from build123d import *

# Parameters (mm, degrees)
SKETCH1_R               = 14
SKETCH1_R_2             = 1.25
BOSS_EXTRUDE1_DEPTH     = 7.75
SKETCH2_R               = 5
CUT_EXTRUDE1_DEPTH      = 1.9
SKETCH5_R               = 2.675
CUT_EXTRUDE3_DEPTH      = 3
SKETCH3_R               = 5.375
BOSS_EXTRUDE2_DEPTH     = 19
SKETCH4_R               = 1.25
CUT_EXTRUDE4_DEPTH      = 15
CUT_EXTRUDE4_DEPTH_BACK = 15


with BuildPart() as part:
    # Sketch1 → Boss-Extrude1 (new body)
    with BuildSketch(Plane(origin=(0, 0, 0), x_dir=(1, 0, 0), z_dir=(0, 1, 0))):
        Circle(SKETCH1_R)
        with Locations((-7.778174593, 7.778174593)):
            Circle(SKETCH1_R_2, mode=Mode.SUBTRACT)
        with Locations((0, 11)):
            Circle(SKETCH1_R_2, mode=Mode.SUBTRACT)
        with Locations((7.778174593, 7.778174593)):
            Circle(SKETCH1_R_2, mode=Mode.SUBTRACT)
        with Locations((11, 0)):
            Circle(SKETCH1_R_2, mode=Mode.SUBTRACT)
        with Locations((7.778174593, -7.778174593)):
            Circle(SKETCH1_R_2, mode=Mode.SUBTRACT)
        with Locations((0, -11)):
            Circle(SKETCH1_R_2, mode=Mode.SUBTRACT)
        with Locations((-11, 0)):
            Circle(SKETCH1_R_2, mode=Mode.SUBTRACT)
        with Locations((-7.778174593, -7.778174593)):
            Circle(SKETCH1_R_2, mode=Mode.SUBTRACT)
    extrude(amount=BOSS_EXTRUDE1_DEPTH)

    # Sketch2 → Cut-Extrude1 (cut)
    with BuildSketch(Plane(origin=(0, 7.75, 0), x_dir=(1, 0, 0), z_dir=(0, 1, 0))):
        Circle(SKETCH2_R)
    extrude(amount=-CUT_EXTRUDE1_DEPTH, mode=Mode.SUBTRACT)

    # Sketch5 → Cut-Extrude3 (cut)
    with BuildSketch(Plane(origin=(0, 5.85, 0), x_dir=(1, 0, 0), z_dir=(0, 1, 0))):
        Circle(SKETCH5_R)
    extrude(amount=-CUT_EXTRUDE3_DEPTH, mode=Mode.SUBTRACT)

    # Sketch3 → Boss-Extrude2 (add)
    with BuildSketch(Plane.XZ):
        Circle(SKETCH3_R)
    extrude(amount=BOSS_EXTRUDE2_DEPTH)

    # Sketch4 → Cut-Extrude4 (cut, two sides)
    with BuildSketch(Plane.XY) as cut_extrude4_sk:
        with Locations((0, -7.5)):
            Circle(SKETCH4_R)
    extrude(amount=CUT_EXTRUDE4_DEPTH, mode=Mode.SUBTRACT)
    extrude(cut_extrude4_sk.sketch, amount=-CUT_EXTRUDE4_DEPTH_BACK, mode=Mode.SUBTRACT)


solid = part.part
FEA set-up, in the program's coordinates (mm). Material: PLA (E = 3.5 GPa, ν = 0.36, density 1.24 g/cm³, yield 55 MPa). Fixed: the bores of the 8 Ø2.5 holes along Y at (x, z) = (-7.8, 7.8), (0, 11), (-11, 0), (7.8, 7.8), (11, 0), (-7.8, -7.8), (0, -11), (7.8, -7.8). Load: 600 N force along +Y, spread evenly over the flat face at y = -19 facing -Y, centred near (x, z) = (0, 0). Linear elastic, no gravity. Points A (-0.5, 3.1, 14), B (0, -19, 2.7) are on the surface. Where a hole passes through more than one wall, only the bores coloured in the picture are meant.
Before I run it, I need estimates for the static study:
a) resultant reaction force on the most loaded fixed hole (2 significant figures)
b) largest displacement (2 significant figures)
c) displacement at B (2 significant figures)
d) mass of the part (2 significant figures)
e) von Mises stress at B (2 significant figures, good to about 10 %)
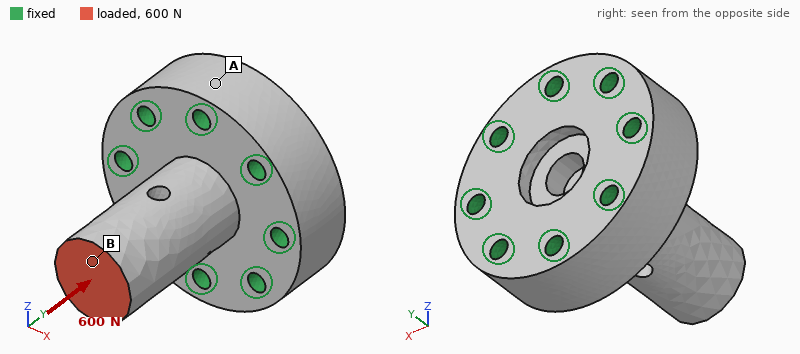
91 N
54 µm
54 µm
7.3 g
6.5 MPa
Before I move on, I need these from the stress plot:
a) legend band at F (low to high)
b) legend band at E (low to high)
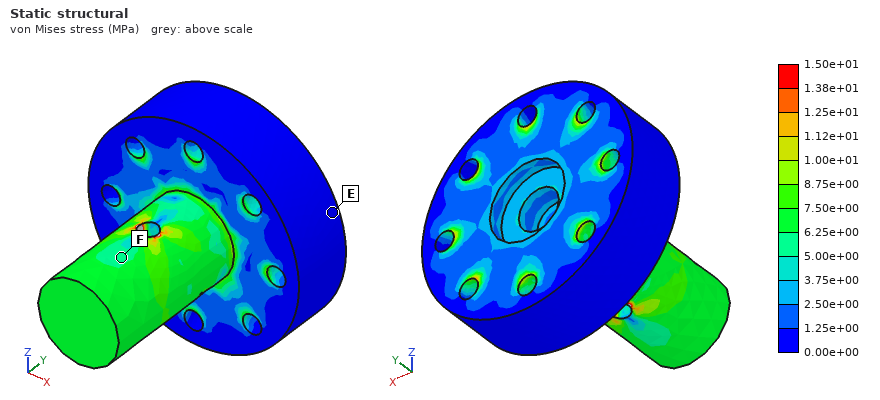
5.00e+00 to 6.25e+00 MPa
0.00e+00 to 1.25e+00 MPa
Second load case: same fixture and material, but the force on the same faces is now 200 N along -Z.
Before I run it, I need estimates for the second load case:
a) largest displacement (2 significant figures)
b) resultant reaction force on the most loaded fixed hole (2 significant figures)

0.39 mm
140 N
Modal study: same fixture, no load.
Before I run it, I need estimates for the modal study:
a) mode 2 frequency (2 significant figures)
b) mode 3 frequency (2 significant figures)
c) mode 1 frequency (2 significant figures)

4800 Hz
12 kHz
4700 Hz
